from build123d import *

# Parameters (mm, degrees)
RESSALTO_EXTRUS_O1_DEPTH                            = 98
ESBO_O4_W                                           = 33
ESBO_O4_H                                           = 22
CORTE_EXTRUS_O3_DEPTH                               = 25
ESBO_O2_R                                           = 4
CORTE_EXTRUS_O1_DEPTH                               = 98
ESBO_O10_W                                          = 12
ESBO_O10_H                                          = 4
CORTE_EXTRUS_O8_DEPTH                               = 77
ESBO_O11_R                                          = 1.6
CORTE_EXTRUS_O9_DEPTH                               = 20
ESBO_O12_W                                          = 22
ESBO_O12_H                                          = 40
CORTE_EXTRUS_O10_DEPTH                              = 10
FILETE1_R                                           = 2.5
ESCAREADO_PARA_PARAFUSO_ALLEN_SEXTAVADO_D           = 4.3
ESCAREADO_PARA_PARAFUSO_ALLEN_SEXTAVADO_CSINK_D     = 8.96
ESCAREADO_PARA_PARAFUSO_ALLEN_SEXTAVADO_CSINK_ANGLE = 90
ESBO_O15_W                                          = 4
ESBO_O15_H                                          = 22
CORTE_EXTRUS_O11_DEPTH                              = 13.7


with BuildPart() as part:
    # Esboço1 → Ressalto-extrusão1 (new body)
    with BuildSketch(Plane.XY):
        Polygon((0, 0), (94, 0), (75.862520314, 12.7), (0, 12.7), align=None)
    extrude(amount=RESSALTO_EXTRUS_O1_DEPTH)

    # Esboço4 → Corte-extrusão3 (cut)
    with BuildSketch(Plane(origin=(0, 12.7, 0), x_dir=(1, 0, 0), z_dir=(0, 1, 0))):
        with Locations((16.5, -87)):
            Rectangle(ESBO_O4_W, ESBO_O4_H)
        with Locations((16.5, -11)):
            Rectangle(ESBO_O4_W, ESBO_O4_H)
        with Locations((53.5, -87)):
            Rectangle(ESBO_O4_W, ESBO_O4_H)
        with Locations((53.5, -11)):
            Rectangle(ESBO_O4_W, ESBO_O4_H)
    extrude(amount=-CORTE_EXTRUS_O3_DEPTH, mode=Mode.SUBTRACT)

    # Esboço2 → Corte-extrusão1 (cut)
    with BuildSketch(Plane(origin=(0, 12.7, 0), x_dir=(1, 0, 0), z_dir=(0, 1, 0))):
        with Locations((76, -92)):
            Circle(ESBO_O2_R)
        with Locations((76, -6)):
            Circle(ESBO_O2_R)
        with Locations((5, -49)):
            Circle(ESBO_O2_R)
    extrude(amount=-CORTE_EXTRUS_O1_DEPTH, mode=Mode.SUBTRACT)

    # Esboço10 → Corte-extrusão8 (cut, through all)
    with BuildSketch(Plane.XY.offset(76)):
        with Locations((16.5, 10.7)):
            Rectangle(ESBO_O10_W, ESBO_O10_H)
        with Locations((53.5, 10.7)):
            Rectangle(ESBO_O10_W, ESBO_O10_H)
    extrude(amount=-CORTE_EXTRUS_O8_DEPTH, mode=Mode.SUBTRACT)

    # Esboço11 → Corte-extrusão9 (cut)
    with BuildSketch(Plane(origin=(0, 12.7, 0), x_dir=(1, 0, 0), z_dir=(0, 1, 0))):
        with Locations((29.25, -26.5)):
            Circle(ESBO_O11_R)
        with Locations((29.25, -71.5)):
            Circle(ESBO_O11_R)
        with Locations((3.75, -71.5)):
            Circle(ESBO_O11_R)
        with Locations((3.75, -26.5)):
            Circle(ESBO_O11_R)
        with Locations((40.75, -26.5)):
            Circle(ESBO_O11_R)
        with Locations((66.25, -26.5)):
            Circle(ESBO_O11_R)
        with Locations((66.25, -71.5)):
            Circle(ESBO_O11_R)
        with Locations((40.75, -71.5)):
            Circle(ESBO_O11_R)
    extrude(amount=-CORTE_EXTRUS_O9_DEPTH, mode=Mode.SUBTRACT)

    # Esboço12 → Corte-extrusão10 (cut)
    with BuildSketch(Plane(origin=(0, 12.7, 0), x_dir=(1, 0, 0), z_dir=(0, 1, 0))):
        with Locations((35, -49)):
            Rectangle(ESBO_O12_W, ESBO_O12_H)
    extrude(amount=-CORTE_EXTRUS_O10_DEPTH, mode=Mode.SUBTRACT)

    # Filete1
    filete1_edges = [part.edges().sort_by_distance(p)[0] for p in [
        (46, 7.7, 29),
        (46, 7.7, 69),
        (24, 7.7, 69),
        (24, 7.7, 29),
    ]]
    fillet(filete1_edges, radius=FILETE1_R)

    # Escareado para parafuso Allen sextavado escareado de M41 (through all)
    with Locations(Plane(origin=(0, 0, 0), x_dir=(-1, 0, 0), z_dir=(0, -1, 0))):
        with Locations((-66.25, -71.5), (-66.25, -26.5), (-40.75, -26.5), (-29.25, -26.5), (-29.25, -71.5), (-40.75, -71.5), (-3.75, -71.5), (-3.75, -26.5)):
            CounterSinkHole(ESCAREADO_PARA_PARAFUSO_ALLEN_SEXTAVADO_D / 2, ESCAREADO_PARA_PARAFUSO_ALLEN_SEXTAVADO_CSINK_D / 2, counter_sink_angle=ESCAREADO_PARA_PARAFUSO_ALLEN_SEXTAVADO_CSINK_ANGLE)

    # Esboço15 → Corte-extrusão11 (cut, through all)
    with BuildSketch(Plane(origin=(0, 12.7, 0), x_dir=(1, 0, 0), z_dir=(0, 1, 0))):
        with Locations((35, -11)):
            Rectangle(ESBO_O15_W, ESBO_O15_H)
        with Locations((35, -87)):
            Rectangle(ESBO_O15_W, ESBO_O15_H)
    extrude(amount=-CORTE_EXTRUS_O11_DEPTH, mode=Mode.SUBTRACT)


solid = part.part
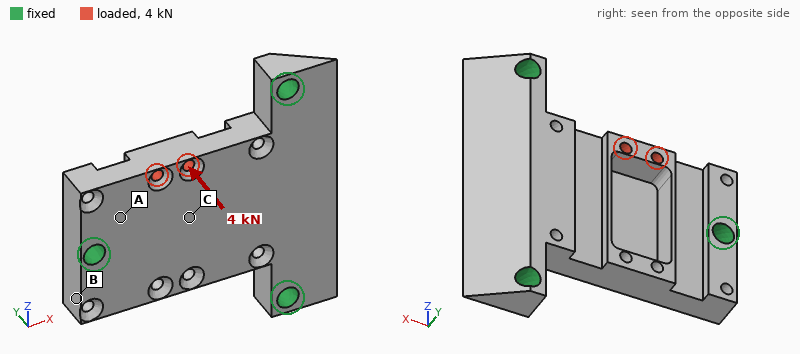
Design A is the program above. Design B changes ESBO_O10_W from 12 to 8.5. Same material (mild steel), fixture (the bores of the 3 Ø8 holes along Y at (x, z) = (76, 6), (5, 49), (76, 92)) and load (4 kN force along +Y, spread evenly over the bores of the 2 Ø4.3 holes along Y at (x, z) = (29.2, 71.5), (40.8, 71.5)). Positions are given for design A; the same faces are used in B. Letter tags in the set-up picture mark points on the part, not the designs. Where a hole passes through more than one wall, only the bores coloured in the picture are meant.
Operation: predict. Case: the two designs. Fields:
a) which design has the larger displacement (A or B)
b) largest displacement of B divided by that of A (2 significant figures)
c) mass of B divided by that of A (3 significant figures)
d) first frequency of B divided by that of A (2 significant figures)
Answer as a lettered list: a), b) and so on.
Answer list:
a) A
b) 0.91
c) 1.03
d) 1.0
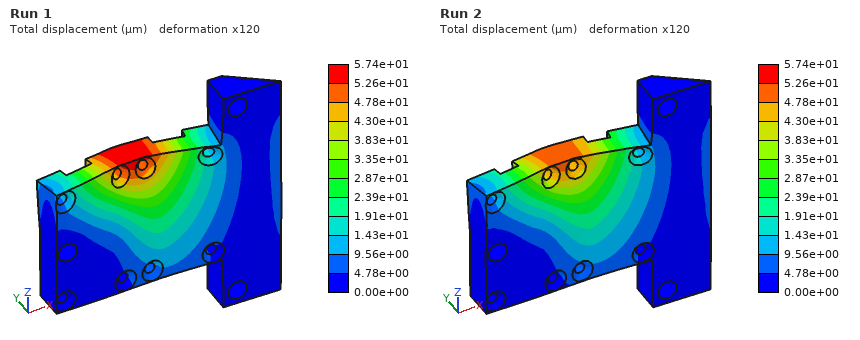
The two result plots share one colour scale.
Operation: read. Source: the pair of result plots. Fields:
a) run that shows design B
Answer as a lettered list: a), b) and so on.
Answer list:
a) Run 2
